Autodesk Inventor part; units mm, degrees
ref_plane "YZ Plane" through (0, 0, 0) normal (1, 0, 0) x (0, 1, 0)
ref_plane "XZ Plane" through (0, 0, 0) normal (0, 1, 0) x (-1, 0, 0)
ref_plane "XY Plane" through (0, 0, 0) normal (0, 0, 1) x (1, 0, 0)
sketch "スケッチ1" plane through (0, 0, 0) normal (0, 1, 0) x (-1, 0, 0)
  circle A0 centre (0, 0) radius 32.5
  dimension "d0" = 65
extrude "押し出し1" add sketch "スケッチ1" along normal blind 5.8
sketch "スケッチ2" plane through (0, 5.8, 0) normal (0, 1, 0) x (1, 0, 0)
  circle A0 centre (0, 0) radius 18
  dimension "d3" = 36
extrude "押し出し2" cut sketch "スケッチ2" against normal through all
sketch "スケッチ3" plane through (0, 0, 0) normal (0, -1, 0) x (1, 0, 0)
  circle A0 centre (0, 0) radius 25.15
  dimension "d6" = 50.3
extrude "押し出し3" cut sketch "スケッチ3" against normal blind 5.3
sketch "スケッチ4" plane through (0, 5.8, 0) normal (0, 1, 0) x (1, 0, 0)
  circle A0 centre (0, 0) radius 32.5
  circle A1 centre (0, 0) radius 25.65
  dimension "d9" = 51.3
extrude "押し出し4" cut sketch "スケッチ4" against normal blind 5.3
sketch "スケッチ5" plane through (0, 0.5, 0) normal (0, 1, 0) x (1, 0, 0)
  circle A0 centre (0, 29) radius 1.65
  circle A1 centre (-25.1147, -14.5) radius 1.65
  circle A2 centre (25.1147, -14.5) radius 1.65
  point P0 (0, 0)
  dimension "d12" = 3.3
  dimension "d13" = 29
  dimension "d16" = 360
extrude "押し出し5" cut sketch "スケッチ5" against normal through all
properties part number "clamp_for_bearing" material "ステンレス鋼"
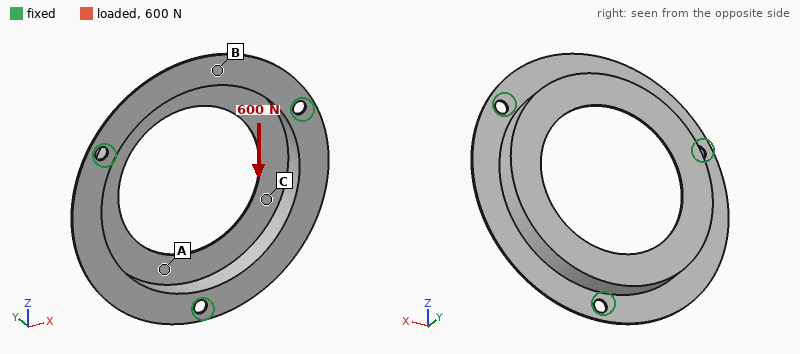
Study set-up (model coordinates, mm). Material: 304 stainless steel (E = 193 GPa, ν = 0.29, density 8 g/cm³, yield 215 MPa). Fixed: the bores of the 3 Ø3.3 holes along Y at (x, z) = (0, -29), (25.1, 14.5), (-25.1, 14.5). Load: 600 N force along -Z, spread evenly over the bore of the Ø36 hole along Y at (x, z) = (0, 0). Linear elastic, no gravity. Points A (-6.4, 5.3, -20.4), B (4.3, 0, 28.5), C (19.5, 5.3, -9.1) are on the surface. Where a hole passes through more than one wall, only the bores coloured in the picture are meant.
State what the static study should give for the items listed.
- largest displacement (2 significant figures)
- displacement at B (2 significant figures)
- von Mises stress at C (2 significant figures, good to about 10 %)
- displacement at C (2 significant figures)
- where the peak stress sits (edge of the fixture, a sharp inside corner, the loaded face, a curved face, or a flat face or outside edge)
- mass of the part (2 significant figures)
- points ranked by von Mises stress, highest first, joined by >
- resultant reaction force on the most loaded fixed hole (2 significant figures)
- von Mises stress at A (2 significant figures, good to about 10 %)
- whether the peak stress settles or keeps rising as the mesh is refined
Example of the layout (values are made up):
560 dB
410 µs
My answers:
62 µm
48 µm
26 MPa
16 µm
edge of the fixture
12 g
A > C > B
210 N
49 MPa
keeps rising
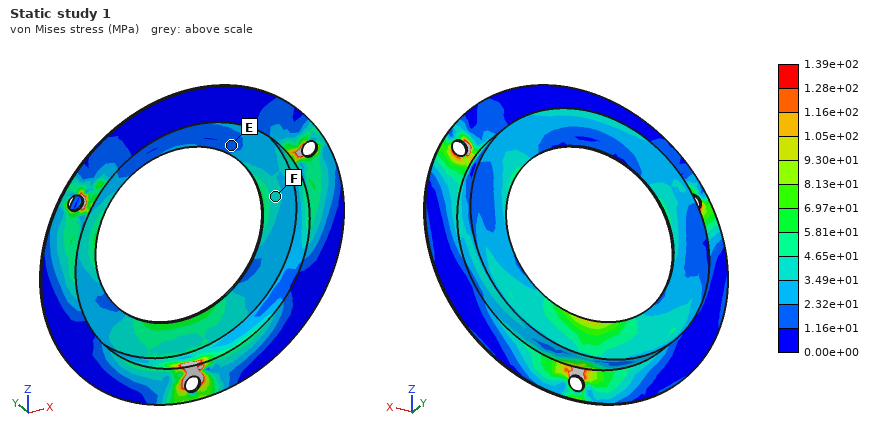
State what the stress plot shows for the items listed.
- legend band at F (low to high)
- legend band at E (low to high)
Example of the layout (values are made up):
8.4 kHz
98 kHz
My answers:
3.49e+01 to 4.65e+01 MPa
1.16e+01 to 2.32e+01 MPa
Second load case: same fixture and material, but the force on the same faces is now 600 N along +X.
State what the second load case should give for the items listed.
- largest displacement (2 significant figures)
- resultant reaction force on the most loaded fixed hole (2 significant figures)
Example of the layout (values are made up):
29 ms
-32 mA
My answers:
54 µm
210 N
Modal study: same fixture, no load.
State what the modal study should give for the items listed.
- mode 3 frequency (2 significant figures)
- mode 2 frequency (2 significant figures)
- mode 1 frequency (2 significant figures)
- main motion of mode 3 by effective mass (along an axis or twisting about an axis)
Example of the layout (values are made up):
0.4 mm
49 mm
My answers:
4600 Hz
3400 Hz
3400 Hz
along Y
